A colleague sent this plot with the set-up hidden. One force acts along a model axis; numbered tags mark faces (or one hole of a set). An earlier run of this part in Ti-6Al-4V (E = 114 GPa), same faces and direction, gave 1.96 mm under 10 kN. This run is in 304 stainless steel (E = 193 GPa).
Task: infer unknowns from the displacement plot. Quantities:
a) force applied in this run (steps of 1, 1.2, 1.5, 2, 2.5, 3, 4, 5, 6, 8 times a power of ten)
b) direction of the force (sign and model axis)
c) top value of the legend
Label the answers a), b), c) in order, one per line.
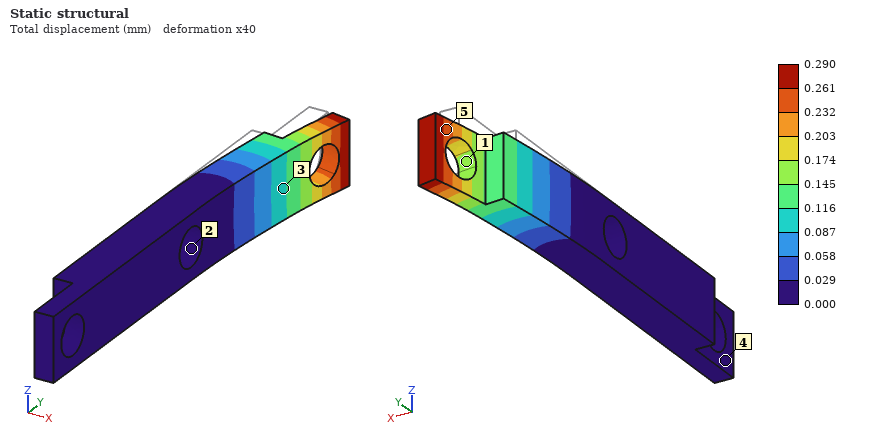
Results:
a) 2.5 kN
b) +X
c) 0.290 mm
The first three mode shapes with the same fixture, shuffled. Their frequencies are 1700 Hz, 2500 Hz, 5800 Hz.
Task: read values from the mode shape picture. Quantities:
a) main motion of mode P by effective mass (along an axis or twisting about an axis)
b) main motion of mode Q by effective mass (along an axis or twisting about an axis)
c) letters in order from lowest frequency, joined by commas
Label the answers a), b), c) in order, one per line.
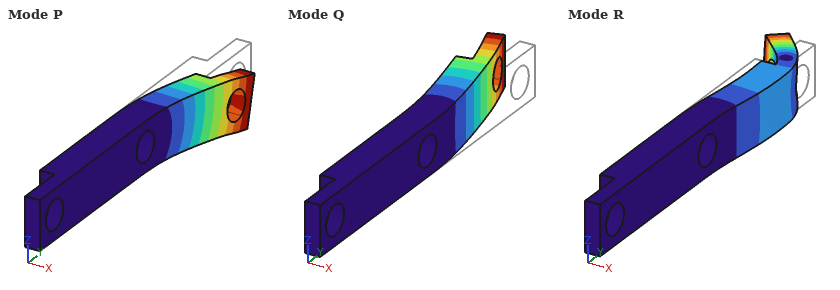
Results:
a) along Z
b) along X
c) Q, P, R
